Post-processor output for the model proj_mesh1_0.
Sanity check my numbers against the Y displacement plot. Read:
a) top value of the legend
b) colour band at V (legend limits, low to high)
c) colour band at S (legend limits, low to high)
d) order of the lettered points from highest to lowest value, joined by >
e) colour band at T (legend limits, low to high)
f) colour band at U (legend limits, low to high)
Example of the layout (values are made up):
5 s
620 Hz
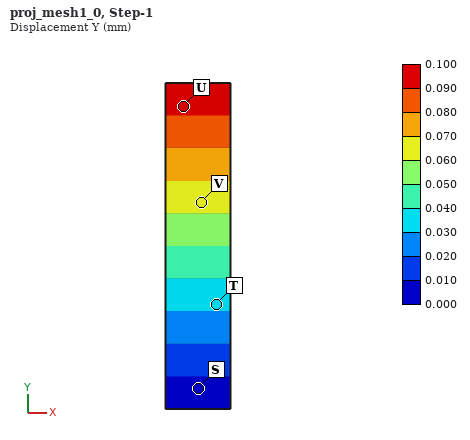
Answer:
0.100 mm
0.060 to 0.070 mm
0.000 to 0.010 mm
U > V > T > S
0.030 to 0.040 mm
0.090 to 0.100 mm
